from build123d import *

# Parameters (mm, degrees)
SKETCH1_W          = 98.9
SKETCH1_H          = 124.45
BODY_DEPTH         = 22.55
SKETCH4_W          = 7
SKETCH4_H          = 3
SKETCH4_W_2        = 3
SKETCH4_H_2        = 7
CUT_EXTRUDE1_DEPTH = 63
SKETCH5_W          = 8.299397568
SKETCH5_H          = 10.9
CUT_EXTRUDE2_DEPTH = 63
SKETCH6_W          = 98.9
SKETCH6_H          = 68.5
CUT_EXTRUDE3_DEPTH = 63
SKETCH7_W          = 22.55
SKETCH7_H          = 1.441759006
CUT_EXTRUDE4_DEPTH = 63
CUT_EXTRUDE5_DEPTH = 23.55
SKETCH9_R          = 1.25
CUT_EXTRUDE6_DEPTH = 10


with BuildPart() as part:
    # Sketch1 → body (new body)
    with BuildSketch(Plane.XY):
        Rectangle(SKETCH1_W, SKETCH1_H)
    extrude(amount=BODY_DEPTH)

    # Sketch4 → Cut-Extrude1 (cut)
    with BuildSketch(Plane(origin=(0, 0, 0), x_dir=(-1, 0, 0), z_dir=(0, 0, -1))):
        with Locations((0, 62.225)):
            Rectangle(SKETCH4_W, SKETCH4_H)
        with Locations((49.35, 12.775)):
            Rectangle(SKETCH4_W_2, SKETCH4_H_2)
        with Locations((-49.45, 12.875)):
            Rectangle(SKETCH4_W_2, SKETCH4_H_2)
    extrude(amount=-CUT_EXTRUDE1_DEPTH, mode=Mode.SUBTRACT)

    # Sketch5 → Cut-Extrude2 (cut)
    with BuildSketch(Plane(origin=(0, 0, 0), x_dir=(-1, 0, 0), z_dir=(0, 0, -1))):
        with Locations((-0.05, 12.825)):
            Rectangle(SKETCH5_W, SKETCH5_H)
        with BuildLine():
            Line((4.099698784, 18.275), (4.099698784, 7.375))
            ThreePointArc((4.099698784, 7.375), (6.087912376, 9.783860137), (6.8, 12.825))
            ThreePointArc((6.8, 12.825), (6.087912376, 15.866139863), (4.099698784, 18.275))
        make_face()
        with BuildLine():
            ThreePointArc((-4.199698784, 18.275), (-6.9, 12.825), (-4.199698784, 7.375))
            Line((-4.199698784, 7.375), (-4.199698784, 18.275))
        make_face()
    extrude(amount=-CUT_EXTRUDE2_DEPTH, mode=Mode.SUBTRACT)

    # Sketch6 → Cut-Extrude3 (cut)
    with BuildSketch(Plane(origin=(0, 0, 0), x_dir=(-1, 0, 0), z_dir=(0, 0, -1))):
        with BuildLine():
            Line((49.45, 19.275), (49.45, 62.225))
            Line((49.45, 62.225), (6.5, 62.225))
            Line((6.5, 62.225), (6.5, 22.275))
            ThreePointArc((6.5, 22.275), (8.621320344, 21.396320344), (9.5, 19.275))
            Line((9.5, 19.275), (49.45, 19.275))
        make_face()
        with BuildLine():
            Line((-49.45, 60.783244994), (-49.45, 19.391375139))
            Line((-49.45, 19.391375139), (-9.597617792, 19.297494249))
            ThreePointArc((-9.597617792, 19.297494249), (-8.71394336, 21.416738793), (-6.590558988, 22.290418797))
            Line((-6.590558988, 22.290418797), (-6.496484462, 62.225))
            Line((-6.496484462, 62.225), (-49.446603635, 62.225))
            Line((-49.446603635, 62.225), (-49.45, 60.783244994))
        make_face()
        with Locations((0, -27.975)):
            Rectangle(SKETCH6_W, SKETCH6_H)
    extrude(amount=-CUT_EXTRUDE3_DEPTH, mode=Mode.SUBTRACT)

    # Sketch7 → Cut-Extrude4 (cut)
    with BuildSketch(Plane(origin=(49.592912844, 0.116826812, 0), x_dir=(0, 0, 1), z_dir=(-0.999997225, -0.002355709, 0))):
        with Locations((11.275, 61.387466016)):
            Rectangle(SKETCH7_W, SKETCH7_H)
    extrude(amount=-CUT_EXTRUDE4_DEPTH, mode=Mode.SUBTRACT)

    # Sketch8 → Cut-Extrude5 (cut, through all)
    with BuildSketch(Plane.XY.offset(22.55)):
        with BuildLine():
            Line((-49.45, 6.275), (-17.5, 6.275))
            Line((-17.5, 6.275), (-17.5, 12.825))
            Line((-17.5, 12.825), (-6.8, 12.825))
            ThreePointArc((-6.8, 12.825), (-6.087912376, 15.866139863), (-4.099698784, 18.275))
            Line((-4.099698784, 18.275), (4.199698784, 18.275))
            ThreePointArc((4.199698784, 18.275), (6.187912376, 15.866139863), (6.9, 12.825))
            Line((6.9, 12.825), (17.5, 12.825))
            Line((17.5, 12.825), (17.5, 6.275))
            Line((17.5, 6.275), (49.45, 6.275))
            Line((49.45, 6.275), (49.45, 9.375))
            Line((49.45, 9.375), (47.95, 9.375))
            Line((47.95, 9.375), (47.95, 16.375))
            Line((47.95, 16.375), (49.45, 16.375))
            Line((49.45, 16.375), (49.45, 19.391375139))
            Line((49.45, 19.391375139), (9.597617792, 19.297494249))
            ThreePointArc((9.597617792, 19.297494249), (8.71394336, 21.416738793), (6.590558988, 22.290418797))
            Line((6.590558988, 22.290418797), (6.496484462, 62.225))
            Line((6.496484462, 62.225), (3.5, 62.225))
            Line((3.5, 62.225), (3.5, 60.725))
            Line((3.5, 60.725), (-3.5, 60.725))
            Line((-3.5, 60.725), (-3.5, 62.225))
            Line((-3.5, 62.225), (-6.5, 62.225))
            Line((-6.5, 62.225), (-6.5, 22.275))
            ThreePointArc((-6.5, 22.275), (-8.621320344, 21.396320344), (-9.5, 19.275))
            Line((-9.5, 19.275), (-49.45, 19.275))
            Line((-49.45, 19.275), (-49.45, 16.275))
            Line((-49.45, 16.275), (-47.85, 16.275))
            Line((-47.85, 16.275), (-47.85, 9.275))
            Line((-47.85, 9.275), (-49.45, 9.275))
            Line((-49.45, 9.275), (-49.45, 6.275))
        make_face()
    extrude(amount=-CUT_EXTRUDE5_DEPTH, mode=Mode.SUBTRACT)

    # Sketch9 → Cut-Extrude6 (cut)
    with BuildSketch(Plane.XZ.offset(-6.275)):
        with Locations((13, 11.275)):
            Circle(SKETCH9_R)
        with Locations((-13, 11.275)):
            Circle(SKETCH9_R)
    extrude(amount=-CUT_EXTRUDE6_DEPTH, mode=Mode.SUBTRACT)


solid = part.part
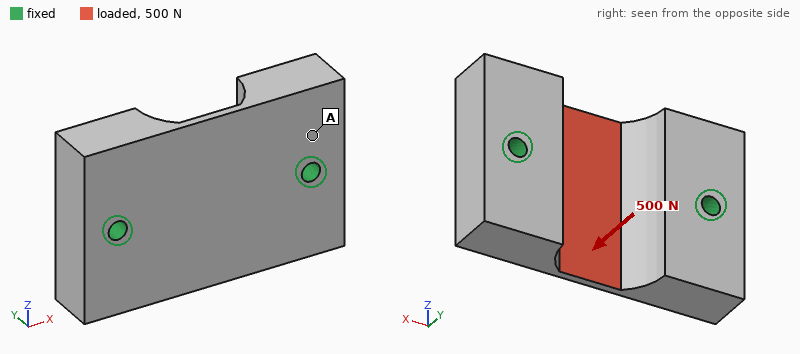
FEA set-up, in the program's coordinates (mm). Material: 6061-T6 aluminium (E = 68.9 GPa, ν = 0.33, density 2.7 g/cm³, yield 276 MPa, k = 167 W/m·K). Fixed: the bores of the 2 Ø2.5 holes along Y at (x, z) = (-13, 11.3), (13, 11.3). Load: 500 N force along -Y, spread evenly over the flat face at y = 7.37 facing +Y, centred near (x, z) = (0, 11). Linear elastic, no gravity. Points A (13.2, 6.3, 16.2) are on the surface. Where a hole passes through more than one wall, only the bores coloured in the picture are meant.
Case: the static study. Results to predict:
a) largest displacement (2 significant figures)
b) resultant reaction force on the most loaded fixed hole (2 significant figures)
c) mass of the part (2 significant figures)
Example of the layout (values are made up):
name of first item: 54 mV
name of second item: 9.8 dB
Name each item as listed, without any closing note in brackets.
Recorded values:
largest displacement: 16 µm
resultant reaction force on the most loaded fixed hole: 360 N
mass of the part: 9.8 g
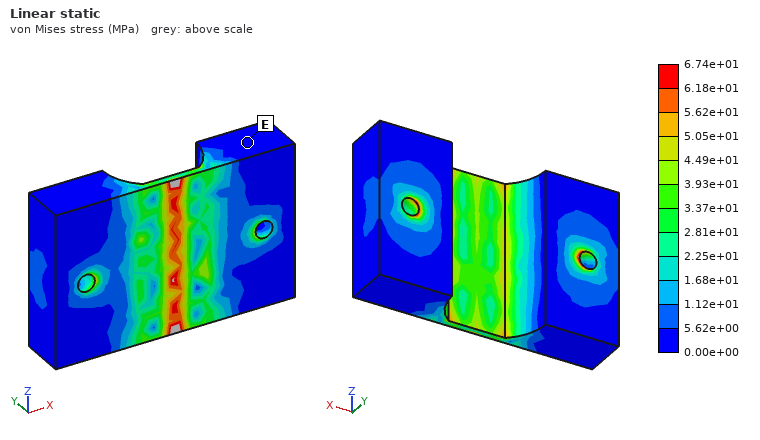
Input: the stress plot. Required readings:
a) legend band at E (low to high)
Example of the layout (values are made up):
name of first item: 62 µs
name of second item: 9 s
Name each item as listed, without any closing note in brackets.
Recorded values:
legend band at E: 0.00e+00 to 5.62e+00 MPa
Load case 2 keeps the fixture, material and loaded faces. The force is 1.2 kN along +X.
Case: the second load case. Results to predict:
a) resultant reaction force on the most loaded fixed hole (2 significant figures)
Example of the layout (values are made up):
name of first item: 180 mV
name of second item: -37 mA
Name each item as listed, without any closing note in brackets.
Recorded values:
resultant reaction force on the most loaded fixed hole: 600 N
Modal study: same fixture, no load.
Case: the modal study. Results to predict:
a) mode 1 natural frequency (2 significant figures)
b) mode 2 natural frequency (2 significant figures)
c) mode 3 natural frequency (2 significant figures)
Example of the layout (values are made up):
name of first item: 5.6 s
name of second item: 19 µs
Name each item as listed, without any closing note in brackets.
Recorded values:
mode 1 natural frequency: 25 kHz
mode 2 natural frequency: 27 kHz
mode 3 natural frequency: 31 kHz
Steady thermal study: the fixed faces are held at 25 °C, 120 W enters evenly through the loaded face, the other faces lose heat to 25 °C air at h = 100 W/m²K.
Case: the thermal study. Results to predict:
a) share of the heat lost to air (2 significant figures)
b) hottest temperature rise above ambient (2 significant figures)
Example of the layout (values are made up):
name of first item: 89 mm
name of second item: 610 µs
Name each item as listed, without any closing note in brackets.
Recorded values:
share of the heat lost to air: 4.1 %
hottest temperature rise above ambient: 83 K
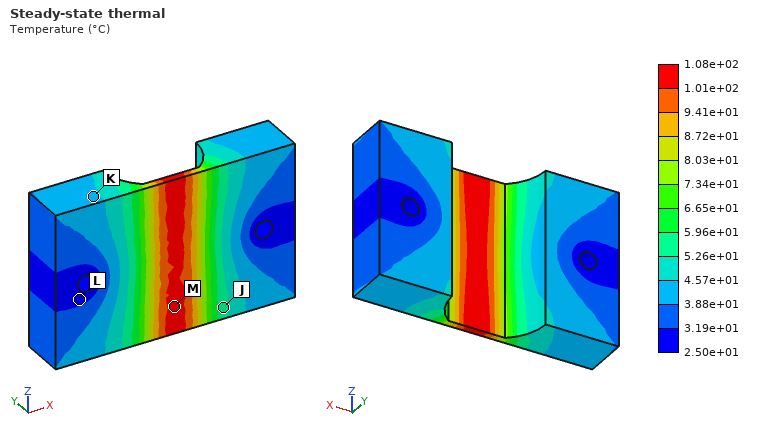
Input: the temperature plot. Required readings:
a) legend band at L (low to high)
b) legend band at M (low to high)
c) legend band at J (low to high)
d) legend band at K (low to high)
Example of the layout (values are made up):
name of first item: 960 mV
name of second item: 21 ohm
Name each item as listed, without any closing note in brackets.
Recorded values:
legend band at L: 2.50e+01 to 3.19e+01 °C
legend band at M: 1.01e+02 to 1.08e+02 °C
legend band at J: 5.26e+01 to 5.96e+01 °C
legend band at K: 3.88e+01 to 4.57e+01 °C
